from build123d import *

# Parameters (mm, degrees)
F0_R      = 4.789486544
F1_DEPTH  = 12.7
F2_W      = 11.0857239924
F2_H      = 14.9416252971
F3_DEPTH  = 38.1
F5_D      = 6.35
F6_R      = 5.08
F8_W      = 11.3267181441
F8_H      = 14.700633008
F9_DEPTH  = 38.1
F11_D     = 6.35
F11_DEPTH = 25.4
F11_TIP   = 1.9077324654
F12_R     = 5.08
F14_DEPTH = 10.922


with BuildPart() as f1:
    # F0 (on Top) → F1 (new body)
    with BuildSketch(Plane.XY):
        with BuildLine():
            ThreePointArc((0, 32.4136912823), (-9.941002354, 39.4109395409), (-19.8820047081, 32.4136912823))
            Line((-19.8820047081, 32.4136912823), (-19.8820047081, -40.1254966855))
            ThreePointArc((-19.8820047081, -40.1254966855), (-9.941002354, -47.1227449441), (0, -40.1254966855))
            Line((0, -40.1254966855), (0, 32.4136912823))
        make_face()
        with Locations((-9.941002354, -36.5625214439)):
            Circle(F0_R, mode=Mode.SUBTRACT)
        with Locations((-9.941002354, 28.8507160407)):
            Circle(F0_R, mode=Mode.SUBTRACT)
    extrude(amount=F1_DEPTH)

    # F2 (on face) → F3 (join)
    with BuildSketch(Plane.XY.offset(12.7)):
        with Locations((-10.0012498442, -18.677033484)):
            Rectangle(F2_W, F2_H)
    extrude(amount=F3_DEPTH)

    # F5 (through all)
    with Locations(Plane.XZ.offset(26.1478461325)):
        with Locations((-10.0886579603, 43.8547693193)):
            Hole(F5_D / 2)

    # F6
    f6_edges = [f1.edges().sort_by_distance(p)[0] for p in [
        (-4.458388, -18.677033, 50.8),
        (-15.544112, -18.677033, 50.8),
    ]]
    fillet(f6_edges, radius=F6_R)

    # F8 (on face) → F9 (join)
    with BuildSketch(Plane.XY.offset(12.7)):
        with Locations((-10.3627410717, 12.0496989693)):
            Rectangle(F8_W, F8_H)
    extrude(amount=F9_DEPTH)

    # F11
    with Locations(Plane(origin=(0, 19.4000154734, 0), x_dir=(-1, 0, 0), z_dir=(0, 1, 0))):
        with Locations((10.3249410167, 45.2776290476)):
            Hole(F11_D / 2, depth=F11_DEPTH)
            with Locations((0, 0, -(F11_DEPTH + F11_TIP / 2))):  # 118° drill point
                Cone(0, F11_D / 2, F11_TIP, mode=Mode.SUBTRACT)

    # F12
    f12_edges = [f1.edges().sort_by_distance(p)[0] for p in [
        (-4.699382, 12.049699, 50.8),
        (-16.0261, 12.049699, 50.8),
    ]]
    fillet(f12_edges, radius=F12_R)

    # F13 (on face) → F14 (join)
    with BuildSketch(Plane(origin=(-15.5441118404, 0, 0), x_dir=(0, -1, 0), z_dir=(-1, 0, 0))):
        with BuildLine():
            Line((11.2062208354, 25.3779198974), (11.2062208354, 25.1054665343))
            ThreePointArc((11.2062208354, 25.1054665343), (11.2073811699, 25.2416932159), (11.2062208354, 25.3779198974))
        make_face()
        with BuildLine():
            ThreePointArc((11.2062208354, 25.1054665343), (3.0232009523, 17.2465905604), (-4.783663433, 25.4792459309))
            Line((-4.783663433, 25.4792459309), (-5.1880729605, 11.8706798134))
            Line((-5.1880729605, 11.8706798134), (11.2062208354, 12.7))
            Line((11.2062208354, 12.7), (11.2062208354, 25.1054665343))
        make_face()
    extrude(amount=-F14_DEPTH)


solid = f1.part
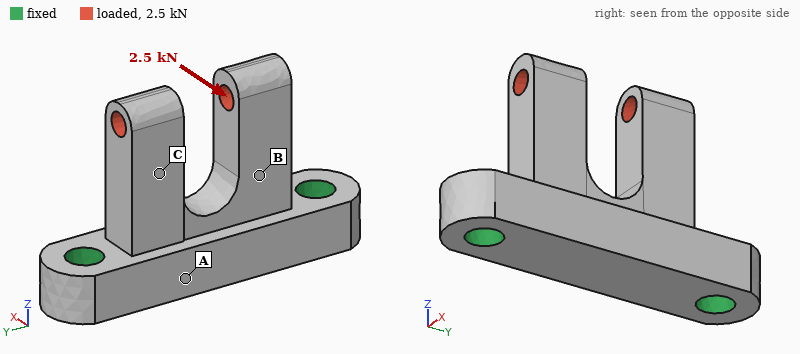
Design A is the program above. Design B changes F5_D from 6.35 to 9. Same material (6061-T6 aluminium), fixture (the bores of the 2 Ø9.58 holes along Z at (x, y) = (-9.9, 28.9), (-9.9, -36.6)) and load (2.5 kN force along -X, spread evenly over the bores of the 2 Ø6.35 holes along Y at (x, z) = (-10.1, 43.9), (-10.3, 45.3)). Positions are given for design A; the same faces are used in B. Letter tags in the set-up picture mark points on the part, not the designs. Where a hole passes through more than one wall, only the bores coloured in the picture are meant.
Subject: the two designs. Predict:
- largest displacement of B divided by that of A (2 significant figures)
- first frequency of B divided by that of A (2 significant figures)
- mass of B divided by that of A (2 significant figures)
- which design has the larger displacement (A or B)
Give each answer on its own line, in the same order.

1.2
1.0
0.98
B
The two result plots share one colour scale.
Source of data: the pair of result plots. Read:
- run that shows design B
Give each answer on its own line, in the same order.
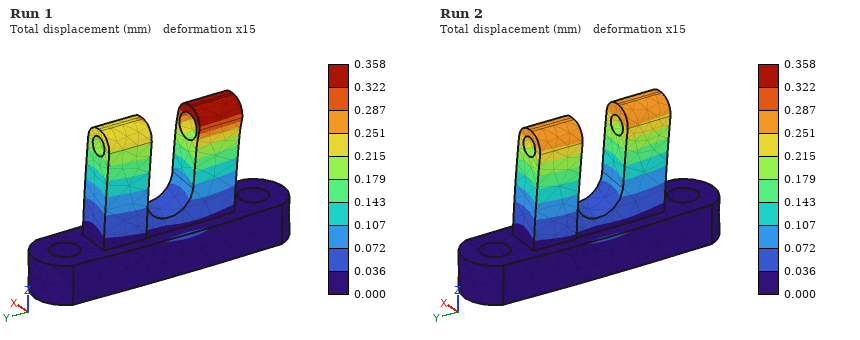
Run 1
